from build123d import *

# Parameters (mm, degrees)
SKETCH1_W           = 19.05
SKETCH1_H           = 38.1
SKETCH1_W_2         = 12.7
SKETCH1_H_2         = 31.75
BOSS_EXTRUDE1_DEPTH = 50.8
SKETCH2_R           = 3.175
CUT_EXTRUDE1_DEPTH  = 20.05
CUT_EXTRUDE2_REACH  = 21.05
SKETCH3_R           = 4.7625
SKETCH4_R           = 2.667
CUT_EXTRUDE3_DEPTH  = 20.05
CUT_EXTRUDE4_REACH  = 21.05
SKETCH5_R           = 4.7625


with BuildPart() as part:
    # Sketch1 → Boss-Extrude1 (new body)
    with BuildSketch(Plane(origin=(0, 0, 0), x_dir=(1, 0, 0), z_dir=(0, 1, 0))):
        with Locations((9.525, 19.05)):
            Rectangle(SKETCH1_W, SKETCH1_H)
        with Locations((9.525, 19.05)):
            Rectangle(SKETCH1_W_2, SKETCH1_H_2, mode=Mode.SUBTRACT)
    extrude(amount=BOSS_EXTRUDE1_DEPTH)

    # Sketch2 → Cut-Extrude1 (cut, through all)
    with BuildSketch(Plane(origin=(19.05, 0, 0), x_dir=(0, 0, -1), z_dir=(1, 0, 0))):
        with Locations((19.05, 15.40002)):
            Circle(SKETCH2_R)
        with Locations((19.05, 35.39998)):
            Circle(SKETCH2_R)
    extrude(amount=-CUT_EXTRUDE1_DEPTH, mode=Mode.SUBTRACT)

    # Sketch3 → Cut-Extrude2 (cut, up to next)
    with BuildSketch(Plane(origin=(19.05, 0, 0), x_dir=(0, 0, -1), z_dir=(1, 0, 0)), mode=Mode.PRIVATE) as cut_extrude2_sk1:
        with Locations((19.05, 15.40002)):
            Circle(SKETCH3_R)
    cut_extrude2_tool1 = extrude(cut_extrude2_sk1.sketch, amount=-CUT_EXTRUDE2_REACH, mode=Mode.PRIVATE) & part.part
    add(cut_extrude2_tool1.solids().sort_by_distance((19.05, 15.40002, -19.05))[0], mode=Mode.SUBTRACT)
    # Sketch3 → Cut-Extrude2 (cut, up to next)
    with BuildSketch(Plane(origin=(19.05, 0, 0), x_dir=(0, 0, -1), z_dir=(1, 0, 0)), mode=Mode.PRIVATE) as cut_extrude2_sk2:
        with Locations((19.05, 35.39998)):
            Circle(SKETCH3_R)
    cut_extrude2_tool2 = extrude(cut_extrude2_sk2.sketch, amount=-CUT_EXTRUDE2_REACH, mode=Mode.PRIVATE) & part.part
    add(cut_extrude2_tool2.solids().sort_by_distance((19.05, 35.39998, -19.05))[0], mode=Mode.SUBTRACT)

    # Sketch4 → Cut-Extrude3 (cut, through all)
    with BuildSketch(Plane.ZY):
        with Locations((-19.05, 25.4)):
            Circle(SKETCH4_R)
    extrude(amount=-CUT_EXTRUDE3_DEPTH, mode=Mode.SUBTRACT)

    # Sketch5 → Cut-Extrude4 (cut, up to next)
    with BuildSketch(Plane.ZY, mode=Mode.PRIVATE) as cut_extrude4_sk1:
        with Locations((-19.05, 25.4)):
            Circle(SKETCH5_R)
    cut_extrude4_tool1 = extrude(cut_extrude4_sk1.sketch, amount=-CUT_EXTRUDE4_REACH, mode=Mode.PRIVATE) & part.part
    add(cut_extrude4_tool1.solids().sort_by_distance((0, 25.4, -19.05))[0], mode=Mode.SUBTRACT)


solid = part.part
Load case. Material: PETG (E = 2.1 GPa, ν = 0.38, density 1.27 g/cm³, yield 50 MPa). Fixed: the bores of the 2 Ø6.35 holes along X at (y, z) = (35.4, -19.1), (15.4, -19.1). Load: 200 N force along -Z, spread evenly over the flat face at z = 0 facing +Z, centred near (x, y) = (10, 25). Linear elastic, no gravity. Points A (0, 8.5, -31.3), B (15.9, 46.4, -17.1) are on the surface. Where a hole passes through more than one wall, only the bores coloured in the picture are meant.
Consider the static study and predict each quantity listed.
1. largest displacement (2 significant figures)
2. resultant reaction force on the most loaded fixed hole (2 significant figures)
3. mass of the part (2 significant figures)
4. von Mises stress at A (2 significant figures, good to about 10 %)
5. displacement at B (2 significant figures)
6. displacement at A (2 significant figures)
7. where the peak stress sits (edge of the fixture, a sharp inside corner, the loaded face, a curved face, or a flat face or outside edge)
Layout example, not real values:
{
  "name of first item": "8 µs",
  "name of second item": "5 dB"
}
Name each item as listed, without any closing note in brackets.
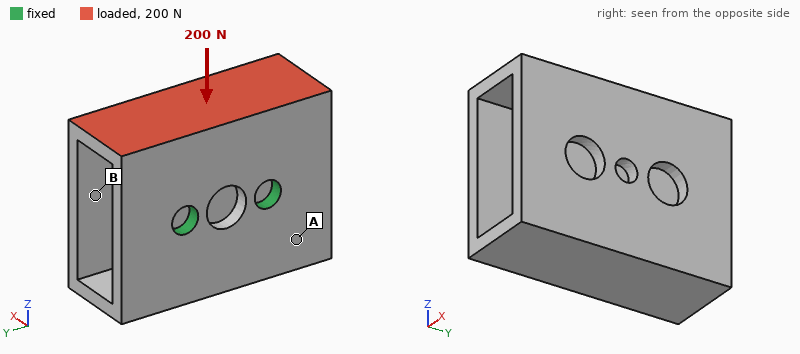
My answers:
{
  "largest displacement": "0.66 mm",
  "resultant reaction force on the most loaded fixed hole": "100 N",
  "mass of the part": "20 g",
  "von Mises stress at A": "4.7 MPa",
  "displacement at B": "0.48 mm",
  "displacement at A": "0.17 mm",
  "where the peak stress sits": "a flat face or outside edge"
}
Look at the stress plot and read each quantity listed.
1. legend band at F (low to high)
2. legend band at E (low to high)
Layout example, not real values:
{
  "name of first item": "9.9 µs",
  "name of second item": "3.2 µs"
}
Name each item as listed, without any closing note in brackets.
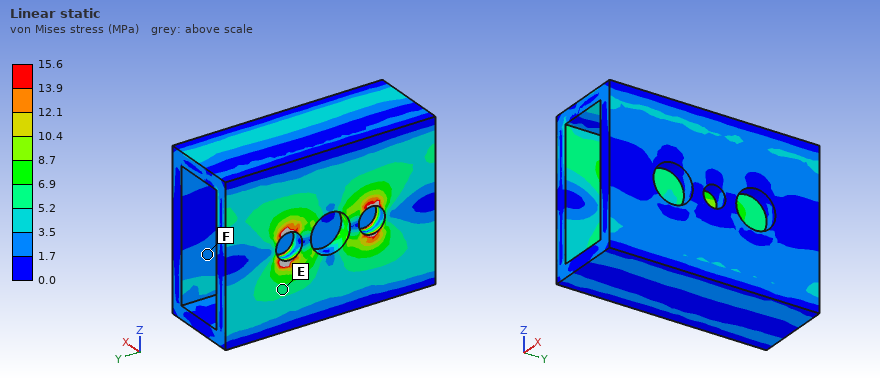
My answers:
{
  "legend band at F": "1.7 to 3.5 MPa",
  "legend band at E": "5.2 to 6.9 MPa"
}
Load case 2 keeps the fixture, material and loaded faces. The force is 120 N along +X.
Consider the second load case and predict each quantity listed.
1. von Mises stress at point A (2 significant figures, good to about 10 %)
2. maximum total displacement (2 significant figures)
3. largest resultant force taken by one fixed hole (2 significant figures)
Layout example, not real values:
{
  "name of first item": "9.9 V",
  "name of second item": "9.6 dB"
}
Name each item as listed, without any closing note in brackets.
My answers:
{
  "von Mises stress at point A": "3.6 MPa",
  "maximum total displacement": "0.70 mm",
  "largest resultant force taken by one fixed hole": "60 N"
}
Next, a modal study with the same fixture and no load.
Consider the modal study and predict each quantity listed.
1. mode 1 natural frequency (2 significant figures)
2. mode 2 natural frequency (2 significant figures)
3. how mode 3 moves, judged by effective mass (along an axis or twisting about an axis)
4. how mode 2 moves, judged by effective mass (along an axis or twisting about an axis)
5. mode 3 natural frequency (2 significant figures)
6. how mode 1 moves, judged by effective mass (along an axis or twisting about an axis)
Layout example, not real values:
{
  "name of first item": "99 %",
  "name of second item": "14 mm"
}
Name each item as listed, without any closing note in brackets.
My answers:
{
  "mode 1 natural frequency": "620 Hz",
  "mode 2 natural frequency": "940 Hz",
  "how mode 3 moves, judged by effective mass": "along X",
  "how mode 2 moves, judged by effective mass": "along Y",
  "mode 3 natural frequency": "1200 Hz",
  "how mode 1 moves, judged by effective mass": "along Z"
}
